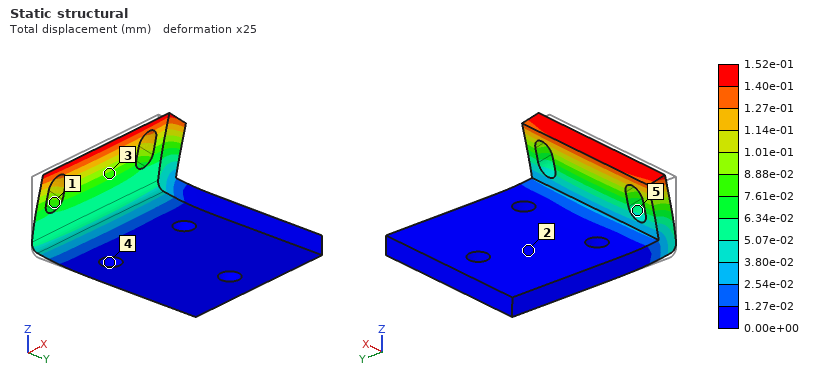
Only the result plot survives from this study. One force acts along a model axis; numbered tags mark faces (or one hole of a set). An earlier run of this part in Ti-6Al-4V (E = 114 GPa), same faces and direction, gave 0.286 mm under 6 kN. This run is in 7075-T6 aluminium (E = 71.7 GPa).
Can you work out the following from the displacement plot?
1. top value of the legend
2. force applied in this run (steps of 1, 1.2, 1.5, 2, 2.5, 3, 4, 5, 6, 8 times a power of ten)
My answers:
1.52e-01 mm
2 kN
